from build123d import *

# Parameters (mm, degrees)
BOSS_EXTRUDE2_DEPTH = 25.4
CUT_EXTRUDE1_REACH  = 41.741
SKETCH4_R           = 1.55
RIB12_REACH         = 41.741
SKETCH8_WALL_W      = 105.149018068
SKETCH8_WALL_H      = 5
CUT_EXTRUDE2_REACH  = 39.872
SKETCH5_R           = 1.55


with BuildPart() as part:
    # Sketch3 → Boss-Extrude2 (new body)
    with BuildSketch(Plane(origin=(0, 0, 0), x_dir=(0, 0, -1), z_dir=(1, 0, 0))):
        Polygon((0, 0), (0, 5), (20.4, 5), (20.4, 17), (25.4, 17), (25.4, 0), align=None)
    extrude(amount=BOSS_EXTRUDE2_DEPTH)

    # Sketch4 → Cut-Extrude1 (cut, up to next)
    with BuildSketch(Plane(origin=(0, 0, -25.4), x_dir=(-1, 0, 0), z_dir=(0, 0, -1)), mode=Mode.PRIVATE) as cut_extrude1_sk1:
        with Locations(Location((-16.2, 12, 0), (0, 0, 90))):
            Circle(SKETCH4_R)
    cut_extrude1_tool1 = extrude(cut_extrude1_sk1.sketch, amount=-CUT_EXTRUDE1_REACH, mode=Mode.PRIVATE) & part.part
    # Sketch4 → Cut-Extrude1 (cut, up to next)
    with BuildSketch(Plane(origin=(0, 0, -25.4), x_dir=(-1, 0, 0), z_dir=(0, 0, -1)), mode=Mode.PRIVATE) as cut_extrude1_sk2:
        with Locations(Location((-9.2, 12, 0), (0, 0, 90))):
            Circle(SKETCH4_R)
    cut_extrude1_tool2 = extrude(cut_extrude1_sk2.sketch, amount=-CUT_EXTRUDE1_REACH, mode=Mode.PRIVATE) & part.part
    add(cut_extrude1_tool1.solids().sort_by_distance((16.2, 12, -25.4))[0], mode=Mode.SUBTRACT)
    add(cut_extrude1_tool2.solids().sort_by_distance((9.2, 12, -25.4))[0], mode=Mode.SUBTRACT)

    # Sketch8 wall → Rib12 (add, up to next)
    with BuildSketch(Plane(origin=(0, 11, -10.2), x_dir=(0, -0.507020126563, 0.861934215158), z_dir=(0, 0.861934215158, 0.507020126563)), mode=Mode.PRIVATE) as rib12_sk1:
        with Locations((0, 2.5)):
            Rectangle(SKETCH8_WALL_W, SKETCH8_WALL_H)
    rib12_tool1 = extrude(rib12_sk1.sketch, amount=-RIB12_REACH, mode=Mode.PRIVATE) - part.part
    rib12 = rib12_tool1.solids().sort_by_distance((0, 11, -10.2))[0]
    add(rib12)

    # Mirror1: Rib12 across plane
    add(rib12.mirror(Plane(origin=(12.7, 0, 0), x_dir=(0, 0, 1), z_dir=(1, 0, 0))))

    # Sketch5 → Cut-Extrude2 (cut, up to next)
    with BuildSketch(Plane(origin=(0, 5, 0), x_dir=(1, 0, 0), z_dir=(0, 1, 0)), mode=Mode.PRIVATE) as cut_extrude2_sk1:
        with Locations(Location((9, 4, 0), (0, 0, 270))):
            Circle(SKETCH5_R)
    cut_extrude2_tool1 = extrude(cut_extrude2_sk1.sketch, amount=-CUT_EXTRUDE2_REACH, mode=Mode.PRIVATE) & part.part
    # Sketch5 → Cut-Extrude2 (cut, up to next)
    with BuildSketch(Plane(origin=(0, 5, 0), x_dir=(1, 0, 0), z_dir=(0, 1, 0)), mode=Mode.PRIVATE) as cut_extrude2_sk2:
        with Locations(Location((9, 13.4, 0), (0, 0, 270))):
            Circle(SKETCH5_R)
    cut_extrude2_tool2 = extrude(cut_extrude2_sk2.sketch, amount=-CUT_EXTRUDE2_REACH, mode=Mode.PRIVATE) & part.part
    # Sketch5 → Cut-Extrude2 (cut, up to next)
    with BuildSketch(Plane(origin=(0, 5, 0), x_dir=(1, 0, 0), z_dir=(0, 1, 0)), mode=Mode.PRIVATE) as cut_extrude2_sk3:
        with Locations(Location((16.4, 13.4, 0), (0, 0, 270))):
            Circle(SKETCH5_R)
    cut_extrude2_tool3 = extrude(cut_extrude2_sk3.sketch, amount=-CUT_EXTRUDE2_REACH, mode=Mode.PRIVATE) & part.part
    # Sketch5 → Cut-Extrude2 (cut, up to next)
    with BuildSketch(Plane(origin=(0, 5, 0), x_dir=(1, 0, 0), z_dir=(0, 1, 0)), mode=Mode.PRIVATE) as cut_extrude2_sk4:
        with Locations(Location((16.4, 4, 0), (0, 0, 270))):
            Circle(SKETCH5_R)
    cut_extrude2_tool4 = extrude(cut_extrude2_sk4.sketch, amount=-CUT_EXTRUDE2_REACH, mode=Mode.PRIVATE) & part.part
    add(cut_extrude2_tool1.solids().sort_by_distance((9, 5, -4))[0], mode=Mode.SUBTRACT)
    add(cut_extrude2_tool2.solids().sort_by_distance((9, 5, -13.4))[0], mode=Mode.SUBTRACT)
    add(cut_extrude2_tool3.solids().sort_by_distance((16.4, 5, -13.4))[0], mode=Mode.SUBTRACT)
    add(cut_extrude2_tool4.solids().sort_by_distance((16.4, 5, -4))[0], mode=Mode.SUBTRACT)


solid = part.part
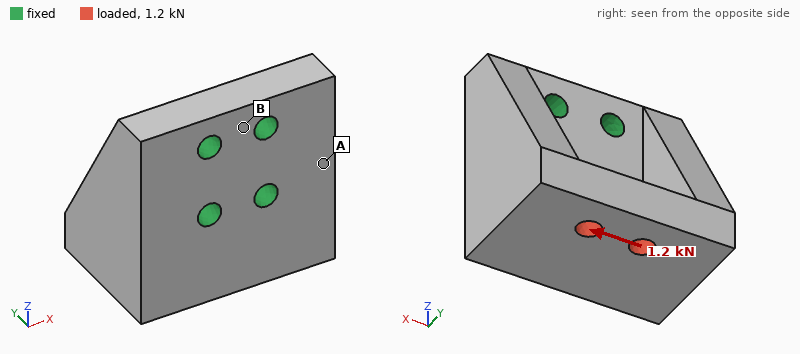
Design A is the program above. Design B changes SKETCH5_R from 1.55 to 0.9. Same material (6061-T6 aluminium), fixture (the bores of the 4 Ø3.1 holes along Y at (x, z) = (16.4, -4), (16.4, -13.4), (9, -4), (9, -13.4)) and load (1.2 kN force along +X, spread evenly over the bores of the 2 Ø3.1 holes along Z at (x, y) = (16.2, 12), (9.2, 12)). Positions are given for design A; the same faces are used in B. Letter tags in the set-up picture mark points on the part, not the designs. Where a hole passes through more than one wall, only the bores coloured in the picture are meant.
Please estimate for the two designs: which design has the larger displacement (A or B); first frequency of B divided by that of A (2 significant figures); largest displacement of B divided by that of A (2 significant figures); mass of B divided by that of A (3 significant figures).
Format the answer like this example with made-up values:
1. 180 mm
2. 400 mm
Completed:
1. B
2. 0.89
3. 1.2
4. 1.02
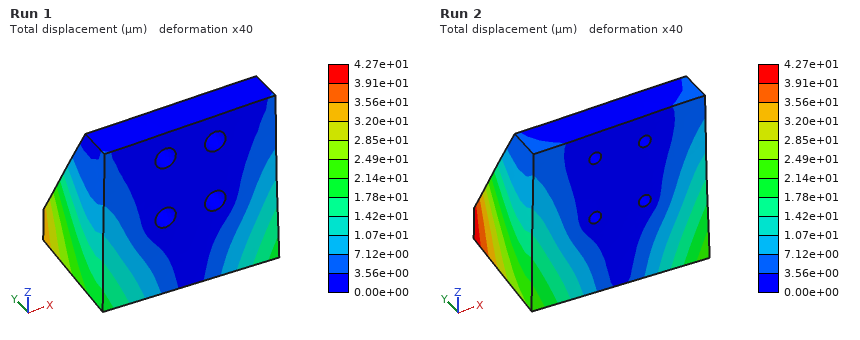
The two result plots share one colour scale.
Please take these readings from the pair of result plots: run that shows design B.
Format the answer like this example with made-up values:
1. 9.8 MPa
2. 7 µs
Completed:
1. Run 2
